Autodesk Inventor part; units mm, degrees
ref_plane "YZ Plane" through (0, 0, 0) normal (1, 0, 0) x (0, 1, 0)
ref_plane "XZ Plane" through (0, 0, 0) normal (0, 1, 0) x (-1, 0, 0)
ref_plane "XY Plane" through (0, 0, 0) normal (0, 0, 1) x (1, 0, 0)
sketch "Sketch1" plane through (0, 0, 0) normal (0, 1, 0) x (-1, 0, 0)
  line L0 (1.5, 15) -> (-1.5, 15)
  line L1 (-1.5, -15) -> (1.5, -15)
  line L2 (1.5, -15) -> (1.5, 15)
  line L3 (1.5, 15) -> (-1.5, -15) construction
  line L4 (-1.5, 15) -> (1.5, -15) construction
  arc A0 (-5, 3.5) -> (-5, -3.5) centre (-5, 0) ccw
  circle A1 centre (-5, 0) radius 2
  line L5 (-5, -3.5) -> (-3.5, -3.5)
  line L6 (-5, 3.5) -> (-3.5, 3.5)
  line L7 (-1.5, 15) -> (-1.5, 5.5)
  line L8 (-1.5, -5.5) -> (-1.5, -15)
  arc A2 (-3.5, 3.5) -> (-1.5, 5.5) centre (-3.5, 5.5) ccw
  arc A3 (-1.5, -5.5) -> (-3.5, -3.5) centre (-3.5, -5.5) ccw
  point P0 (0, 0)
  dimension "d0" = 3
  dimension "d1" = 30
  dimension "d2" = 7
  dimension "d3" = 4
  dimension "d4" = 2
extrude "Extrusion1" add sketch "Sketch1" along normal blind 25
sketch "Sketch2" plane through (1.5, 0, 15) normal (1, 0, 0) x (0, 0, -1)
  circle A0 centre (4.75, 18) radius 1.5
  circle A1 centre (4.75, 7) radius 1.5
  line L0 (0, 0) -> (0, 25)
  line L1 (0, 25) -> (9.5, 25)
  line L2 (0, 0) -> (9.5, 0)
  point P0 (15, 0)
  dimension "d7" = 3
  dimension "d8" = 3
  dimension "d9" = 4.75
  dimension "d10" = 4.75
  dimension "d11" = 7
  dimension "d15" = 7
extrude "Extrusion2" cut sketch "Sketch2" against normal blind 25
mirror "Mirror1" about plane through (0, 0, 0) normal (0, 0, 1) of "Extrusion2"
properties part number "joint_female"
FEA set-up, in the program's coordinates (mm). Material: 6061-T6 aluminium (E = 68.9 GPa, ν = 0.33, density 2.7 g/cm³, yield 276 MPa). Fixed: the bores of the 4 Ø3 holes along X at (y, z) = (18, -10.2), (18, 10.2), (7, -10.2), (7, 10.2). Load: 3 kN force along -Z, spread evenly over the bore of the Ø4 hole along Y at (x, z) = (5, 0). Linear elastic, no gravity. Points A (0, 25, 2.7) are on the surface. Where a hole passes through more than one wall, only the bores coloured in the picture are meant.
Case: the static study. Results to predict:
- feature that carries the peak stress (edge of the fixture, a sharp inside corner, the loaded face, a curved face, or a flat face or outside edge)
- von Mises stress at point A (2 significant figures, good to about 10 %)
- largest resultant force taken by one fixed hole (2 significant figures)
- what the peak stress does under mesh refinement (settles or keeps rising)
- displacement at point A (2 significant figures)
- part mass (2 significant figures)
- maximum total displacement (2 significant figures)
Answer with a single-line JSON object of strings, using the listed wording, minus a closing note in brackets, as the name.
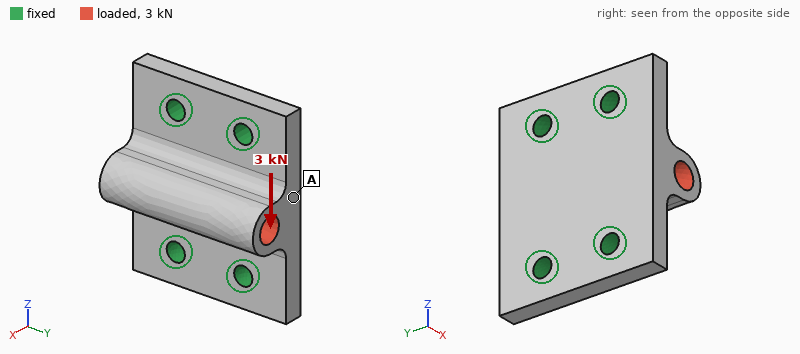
{"feature that carries the peak stress": "edge of the fixture", "von Mises stress at point A": "25 MPa", "largest resultant force taken by one fixed hole": "900 N", "what the peak stress does under mesh refinement": "keeps rising", "displacement at point A": "5.2 µm", "part mass": "8.1 g", "maximum total displacement": "25 µm"}
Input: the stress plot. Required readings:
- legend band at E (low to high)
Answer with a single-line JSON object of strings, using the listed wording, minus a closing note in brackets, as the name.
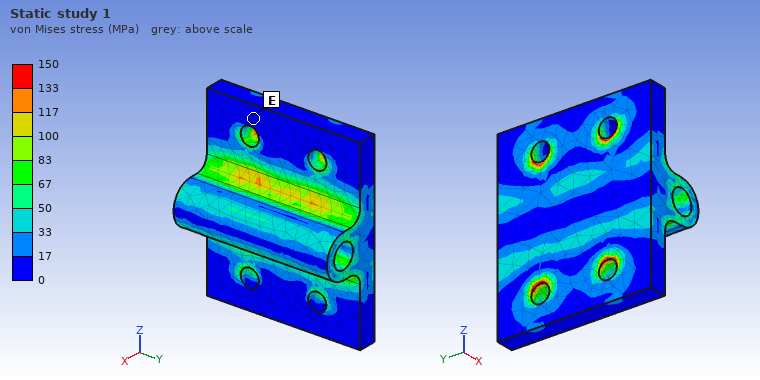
{"legend band at E": "0 to 17 MPa"}
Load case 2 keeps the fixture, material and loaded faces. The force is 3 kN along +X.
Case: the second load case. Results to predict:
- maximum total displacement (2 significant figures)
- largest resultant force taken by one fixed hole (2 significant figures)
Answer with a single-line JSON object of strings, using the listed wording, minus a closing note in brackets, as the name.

{"maximum total displacement": "24 µm", "largest resultant force taken by one fixed hole": "810 N"}
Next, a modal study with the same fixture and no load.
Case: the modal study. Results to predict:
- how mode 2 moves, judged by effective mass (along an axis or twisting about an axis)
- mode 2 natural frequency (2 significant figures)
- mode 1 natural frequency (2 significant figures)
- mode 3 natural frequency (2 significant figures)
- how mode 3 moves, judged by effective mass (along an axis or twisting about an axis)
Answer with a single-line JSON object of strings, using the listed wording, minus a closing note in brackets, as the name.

{"how mode 2 moves, judged by effective mass": "along X", "mode 2 natural frequency": "29 kHz", "mode 1 natural frequency": "24 kHz", "mode 3 natural frequency": "42 kHz", "how mode 3 moves, judged by effective mass": "along Z"}
